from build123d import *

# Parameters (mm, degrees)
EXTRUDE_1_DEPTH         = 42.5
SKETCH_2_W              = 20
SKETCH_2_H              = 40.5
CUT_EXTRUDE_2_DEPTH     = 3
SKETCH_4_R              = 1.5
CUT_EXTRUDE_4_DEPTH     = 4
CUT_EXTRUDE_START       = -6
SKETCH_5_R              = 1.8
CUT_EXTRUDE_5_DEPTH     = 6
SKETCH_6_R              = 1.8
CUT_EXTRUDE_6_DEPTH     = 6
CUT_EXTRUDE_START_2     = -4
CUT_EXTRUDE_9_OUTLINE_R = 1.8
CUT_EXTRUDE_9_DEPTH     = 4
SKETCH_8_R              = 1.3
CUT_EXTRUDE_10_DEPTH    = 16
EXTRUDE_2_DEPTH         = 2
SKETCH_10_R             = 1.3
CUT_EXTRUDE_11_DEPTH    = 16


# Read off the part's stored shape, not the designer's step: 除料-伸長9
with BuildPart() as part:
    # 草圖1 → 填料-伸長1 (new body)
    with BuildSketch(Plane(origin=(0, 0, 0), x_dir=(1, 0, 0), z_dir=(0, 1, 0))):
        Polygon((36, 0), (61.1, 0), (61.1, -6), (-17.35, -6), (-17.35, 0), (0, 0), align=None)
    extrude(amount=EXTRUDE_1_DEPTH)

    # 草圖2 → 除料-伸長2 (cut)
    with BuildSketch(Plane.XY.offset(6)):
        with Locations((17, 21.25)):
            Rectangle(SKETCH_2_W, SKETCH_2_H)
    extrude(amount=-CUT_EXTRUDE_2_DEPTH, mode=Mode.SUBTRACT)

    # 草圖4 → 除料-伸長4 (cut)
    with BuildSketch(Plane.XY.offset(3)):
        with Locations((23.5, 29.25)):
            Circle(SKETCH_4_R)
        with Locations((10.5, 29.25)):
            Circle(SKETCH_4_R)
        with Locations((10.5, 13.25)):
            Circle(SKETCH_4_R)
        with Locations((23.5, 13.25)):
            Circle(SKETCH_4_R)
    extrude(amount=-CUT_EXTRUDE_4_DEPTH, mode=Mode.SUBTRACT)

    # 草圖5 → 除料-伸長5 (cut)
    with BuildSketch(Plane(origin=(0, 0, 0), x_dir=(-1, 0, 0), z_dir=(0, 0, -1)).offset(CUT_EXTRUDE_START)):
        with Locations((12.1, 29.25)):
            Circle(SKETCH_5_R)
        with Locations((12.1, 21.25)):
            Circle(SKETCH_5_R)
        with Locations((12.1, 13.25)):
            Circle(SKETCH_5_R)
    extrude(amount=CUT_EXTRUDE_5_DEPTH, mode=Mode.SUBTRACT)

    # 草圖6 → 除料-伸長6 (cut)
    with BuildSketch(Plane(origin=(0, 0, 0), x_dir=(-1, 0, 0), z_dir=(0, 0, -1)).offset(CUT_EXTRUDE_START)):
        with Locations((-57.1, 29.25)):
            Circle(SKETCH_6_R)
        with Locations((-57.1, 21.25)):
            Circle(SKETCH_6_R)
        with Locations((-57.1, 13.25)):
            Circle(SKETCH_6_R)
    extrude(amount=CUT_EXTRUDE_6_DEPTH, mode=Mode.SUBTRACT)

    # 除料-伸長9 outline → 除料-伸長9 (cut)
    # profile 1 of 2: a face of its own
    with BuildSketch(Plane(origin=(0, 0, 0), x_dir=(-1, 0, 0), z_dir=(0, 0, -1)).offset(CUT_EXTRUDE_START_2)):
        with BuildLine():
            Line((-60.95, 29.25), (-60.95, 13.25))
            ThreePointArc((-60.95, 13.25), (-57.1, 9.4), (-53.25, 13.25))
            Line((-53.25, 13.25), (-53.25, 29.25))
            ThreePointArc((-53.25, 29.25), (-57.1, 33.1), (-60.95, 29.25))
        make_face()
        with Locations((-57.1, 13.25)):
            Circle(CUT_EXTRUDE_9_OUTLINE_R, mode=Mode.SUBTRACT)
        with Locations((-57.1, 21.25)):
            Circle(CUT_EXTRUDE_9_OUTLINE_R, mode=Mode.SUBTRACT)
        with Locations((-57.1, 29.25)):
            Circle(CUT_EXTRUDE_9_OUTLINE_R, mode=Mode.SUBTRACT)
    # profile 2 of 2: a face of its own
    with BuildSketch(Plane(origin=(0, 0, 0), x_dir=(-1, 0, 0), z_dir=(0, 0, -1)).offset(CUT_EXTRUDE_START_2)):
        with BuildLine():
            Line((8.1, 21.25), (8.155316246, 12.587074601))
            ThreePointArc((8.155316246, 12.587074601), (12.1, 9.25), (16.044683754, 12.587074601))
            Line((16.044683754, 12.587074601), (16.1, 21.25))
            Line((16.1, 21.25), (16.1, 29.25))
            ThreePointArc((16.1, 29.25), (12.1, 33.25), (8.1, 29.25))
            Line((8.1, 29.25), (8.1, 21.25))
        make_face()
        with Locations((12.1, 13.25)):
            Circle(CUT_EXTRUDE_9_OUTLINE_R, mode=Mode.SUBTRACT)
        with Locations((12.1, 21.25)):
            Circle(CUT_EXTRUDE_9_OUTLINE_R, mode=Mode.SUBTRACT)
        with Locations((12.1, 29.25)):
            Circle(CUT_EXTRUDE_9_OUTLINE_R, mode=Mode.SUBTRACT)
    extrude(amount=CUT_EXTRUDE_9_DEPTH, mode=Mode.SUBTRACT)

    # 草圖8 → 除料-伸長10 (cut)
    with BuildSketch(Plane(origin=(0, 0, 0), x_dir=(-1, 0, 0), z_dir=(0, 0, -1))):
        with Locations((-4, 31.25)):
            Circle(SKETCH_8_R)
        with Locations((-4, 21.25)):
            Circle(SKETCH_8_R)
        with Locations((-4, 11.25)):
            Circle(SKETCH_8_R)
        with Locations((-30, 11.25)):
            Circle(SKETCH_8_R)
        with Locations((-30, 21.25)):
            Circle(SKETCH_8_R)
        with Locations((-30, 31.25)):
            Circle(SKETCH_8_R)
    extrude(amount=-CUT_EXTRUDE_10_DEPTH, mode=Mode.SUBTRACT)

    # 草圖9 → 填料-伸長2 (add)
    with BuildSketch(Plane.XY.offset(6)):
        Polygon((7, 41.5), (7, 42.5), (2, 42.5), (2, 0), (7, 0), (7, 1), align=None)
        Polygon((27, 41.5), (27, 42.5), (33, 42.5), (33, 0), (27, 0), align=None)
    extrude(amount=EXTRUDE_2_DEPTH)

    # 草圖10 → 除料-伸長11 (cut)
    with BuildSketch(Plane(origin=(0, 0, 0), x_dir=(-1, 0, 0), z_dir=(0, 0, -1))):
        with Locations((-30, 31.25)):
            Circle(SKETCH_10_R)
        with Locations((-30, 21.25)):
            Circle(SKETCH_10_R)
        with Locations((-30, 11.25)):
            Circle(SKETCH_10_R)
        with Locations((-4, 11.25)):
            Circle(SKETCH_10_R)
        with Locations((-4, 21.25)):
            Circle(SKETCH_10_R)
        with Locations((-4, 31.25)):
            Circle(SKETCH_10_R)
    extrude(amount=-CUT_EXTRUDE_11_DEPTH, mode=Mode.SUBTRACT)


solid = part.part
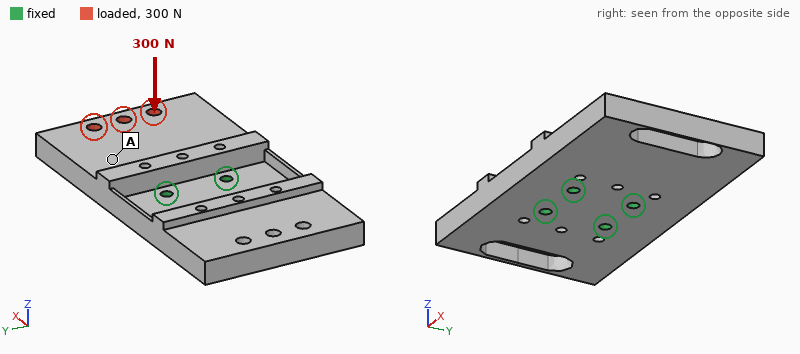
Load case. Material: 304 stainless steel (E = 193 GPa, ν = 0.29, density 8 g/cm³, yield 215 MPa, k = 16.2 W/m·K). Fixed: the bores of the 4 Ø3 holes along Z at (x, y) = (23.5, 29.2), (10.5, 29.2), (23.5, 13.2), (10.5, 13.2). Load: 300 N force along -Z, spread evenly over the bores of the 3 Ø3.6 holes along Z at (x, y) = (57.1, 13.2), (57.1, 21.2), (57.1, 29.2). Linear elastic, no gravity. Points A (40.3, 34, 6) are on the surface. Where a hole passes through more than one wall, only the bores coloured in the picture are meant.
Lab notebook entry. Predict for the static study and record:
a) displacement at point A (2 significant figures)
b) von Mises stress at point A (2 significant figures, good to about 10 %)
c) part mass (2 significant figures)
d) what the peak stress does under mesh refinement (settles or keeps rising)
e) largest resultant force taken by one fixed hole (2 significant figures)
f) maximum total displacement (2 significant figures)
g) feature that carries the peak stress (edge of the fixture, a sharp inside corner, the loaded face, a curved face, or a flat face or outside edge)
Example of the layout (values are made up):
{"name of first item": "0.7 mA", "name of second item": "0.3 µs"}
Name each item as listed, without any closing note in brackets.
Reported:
{"displacement at point A": "0.038 mm", "von Mises stress at point A": "20 MPa", "part mass": "130 g", "what the peak stress does under mesh refinement": "keeps rising", "largest resultant force taken by one fixed hole": "340 N", "maximum total displacement": "0.10 mm", "feature that carries the peak stress": "edge of the fixture"}
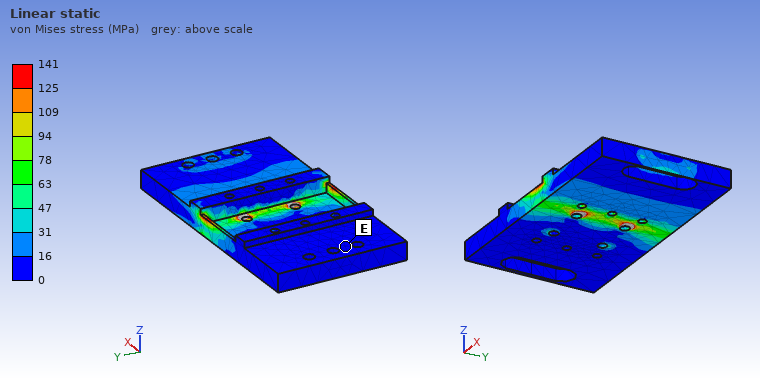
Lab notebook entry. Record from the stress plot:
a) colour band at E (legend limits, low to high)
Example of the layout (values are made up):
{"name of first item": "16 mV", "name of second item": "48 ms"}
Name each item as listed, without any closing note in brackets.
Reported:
{"colour band at E": "0 to 16 MPa"}
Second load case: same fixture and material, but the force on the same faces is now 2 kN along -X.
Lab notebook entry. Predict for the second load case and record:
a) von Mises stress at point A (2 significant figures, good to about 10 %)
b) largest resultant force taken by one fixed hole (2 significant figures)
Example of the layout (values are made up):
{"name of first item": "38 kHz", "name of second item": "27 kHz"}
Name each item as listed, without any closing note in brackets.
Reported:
{"von Mises stress at point A": "23 MPa", "largest resultant force taken by one fixed hole": "760 N"}
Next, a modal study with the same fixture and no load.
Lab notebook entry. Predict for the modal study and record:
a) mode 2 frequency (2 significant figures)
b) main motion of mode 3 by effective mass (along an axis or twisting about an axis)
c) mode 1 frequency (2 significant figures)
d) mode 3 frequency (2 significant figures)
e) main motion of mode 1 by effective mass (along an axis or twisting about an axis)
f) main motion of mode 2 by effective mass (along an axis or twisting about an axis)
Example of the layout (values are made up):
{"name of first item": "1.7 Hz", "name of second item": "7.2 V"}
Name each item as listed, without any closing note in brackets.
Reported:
{"mode 2 frequency": "3200 Hz", "main motion of mode 3 by effective mass": "twisting about X", "mode 1 frequency": "1900 Hz", "mode 3 frequency": "4800 Hz", "main motion of mode 1 by effective mass": "along Z", "main motion of mode 2 by effective mass": "along Z"}
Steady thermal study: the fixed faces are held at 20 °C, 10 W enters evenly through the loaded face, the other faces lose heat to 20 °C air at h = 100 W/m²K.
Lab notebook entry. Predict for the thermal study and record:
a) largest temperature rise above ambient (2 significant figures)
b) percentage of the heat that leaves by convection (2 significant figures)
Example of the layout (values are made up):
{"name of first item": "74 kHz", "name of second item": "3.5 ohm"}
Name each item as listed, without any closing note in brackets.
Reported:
{"largest temperature rise above ambient": "79 K", "percentage of the heat that leaves by convection": "85 %"}
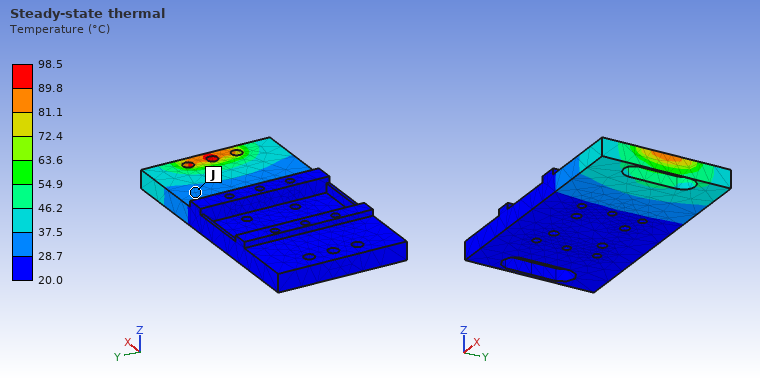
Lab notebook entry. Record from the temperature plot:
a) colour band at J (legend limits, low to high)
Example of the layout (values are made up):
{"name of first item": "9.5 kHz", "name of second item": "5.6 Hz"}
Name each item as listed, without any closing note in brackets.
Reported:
{"colour band at J": "28.7 to 37.5 °C"}
